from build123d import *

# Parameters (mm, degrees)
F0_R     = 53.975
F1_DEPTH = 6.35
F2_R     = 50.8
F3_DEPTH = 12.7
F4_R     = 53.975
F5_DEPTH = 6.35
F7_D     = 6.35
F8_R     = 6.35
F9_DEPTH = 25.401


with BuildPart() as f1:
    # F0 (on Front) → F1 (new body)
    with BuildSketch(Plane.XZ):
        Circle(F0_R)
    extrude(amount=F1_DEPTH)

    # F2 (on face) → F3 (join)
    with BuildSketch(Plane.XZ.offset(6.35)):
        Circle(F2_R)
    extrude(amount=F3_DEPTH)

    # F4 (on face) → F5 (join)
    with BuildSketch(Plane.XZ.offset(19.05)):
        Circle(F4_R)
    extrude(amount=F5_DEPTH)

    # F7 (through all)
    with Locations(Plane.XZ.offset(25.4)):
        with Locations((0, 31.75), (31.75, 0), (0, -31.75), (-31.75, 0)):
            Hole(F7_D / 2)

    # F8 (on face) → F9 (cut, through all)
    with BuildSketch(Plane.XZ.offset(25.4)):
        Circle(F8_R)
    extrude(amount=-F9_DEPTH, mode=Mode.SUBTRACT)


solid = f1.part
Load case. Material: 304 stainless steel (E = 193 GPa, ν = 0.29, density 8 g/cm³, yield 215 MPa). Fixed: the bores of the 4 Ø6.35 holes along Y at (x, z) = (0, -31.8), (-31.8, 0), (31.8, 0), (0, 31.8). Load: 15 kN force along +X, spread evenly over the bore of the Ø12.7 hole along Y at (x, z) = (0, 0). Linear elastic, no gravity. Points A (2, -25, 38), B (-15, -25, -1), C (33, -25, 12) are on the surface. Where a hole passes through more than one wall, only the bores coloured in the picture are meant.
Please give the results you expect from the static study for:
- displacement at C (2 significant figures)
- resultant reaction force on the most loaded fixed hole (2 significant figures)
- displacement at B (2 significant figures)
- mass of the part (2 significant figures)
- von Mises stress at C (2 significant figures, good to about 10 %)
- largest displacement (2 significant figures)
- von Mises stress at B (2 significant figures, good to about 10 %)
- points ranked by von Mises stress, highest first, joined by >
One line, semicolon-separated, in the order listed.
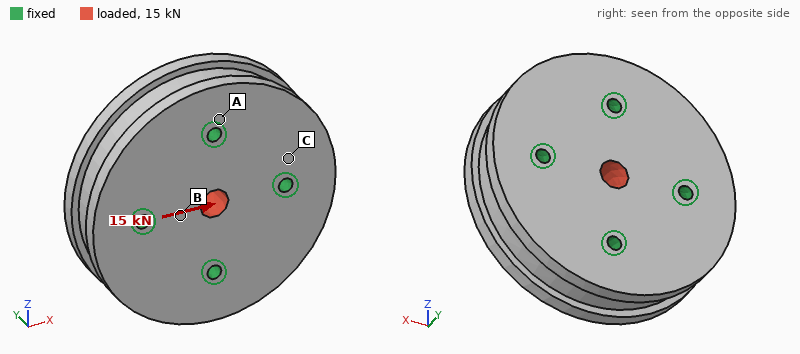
0.36 µm; 4.9 kN; 0.91 µm; 1.7 kg; 3.6 MPa; 1.6 µm; 13 MPa; B > C > A
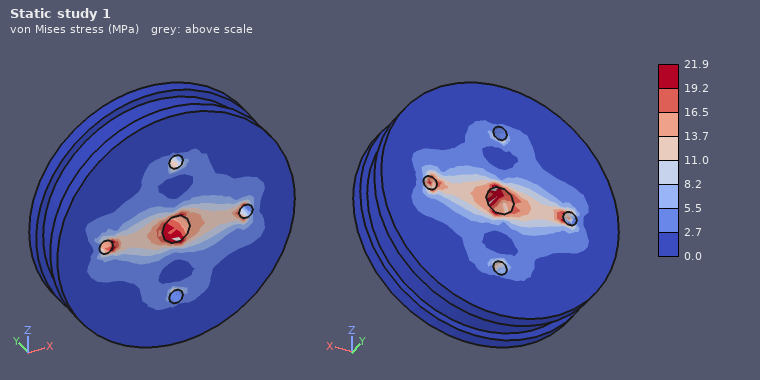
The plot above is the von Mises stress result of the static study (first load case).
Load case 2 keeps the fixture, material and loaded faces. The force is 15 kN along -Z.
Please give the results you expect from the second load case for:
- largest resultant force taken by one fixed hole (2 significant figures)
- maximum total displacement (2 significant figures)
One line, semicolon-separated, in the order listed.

4.9 kN; 1.6 µm
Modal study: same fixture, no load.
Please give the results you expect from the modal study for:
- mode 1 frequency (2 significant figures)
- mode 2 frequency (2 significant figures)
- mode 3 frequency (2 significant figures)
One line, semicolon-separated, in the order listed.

14 kHz; 15 kHz; 15 kHz
